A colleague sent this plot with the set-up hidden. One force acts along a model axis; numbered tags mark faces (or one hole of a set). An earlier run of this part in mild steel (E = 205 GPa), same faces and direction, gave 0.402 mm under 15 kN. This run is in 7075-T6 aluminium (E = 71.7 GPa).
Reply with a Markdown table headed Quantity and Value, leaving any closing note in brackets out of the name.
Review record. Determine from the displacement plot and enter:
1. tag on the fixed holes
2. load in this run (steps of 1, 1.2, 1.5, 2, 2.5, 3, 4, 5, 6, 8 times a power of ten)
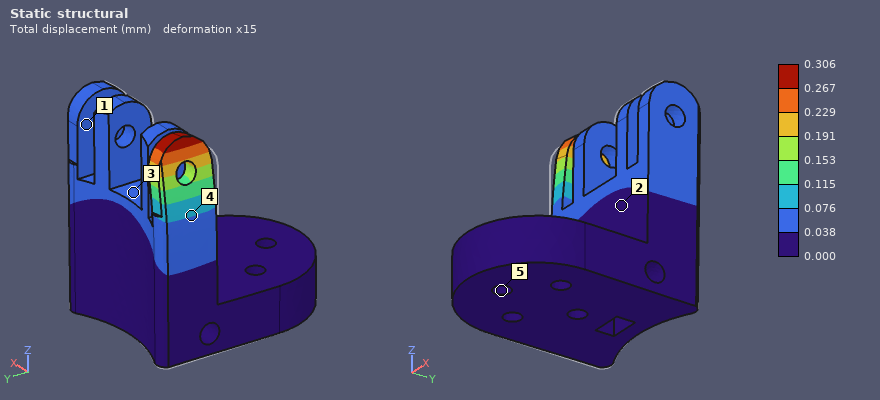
| Quantity | Value |
|---|---|
| tag on the fixed holes | 5 |
| load in this run | 4 kN |
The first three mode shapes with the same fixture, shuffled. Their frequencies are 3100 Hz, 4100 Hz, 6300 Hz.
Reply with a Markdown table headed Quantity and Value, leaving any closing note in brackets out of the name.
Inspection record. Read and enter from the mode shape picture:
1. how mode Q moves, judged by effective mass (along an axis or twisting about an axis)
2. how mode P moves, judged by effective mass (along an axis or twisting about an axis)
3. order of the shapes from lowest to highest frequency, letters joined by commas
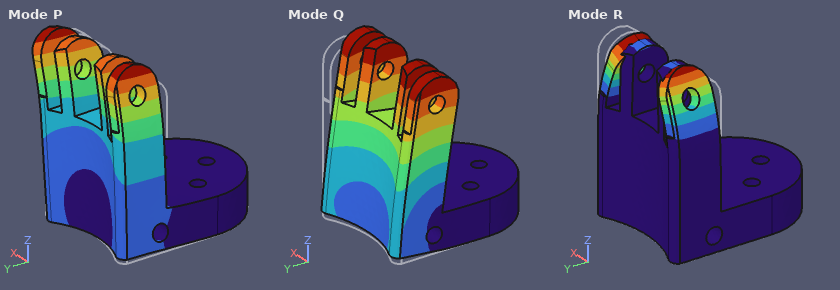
| Quantity | Value |
|---|---|
| how mode Q moves, judged by effective mass | along Y |
| how mode P moves, judged by effective mass | along X |
| order of the shapes from lowest to highest frequency, letters joined by commas | Q, P, R |
